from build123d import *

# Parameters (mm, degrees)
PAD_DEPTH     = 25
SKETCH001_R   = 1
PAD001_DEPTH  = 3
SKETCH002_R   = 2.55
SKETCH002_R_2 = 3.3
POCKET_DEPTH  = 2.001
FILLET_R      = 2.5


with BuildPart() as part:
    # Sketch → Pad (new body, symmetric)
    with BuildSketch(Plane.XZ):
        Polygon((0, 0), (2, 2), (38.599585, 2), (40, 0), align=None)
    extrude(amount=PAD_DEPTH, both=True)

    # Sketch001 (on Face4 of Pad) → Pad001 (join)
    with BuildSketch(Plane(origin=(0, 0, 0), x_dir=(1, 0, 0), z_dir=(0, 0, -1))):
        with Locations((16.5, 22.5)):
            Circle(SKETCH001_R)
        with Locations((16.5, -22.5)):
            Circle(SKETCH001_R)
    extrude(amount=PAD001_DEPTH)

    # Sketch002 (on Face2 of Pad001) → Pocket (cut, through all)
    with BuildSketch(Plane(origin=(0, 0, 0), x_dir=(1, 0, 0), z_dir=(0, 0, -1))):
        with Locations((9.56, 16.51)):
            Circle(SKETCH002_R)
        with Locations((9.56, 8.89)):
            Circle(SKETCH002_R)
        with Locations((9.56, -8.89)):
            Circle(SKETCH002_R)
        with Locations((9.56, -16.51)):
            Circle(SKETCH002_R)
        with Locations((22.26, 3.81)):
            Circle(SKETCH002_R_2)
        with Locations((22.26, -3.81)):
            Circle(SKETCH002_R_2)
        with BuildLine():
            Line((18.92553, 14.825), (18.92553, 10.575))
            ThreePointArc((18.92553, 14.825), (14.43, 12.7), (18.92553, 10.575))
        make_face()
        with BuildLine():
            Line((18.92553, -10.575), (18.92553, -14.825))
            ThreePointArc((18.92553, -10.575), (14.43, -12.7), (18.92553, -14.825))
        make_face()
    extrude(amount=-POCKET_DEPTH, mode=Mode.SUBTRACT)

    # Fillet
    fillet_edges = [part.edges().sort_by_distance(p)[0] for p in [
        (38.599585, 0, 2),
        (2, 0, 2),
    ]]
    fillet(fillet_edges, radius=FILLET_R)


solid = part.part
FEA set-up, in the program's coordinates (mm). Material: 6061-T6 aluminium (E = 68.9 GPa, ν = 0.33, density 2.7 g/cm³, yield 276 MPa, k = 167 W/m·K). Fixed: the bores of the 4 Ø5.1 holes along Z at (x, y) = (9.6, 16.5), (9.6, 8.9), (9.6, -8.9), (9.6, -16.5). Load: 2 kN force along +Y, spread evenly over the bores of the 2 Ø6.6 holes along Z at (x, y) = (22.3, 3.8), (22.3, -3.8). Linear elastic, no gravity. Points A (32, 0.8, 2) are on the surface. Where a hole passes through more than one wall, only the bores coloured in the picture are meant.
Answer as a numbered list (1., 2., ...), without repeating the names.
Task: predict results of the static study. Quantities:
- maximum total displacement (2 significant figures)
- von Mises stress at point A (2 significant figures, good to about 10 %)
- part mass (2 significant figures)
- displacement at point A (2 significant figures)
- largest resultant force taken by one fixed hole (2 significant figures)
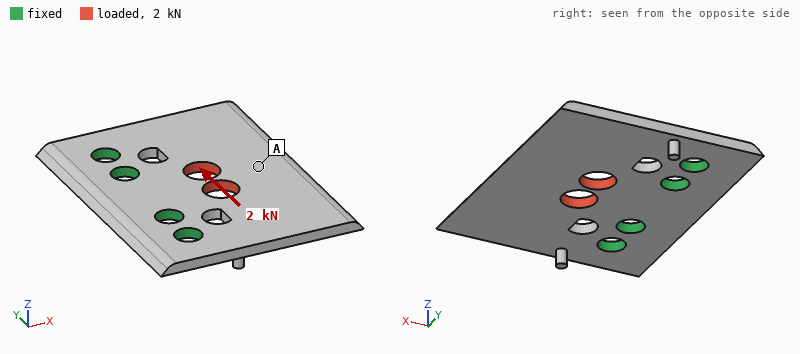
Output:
1. 31 µm
2. 17 MPa
3. 9.3 g
4. 22 µm
5. 650 N
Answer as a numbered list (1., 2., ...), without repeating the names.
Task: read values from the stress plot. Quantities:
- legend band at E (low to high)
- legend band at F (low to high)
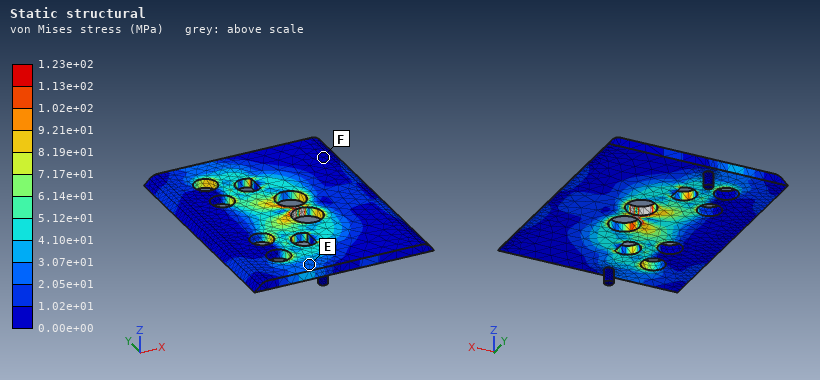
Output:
1. 2.05e+01 to 3.07e+01 MPa
2. 0.00e+00 to 1.02e+01 MPa
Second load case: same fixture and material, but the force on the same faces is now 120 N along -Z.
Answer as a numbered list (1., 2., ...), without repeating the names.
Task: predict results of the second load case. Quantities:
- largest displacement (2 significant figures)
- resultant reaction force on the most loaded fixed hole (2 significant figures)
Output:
1. 0.11 mm
2. 55 N
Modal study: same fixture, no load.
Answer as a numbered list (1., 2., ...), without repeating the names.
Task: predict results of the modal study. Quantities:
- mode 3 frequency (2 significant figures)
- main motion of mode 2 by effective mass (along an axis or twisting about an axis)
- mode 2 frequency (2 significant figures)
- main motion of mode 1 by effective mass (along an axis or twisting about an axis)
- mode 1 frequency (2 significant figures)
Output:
1. 6500 Hz
2. twisting about X
3. 3100 Hz
4. along Z
5. 1900 Hz
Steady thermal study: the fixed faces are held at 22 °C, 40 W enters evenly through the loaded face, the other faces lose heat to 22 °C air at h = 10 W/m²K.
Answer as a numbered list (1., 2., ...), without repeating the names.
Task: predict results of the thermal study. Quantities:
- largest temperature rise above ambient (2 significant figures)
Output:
1. 64 K
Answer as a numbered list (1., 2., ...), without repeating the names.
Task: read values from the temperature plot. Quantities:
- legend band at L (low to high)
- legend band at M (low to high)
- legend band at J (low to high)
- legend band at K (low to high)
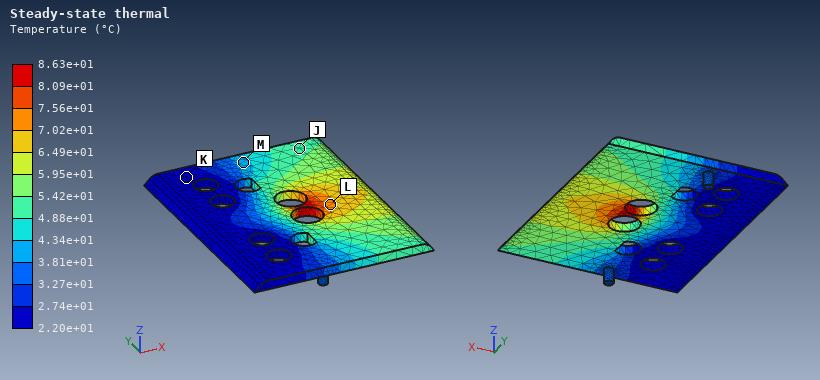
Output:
1. 7.02e+01 to 7.56e+01 °C
2. 3.81e+01 to 4.34e+01 °C
3. 4.88e+01 to 5.42e+01 °C
4. 2.20e+01 to 2.74e+01 °C
